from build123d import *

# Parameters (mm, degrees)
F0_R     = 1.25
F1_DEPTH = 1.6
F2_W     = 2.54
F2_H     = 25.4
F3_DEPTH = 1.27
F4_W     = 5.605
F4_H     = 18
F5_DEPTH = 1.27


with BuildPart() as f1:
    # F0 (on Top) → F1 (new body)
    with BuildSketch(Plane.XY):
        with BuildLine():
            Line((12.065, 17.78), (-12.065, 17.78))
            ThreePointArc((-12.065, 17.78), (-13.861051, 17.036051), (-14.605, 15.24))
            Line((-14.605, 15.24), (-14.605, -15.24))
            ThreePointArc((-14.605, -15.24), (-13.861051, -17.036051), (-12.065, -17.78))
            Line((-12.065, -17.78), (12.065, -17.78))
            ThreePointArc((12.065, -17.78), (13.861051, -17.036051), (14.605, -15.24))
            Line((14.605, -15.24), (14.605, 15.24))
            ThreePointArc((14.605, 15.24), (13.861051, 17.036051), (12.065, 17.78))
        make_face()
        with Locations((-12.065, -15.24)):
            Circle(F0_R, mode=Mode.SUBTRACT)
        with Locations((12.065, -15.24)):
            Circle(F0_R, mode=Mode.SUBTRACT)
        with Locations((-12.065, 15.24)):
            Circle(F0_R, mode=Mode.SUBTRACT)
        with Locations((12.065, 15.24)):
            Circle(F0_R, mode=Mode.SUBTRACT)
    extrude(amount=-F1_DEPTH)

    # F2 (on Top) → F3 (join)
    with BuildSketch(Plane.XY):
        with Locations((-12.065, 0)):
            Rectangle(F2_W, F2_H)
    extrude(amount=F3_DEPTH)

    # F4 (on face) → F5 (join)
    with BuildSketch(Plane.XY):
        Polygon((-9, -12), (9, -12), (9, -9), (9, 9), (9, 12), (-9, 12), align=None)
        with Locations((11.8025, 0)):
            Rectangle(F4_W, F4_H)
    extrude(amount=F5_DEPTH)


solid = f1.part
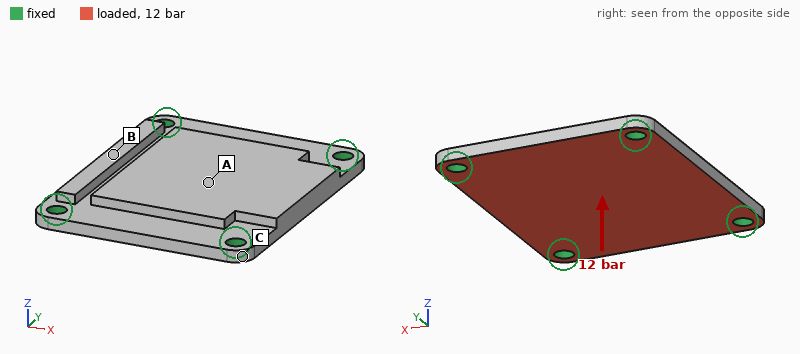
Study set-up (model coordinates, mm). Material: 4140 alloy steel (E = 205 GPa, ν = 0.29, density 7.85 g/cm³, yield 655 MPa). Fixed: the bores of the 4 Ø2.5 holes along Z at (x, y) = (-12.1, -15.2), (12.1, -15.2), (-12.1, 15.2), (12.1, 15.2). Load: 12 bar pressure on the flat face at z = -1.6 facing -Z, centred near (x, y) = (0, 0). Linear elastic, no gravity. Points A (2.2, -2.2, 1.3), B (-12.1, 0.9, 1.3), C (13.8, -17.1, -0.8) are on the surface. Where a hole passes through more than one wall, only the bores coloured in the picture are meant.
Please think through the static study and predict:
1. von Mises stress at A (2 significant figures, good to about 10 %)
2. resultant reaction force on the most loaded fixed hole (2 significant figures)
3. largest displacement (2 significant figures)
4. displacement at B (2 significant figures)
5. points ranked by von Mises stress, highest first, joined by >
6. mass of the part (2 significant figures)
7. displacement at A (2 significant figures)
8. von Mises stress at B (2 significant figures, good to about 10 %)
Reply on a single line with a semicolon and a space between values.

48 MPa; 400 N; 22 µm; 19 µm; B > A > C; 19 g; 21 µm; 93 MPa
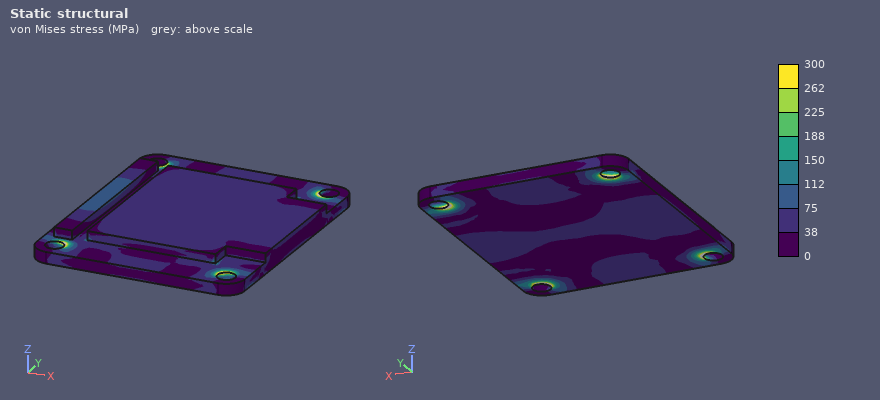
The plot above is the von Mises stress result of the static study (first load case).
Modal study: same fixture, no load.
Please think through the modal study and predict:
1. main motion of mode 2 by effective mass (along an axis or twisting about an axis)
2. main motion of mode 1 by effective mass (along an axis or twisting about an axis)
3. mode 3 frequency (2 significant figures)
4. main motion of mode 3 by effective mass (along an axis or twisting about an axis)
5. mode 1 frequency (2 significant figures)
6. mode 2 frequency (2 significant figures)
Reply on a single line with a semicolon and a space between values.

twisting about Y; along Z; 18 kHz; twisting about X; 9400 Hz; 14 kHz
